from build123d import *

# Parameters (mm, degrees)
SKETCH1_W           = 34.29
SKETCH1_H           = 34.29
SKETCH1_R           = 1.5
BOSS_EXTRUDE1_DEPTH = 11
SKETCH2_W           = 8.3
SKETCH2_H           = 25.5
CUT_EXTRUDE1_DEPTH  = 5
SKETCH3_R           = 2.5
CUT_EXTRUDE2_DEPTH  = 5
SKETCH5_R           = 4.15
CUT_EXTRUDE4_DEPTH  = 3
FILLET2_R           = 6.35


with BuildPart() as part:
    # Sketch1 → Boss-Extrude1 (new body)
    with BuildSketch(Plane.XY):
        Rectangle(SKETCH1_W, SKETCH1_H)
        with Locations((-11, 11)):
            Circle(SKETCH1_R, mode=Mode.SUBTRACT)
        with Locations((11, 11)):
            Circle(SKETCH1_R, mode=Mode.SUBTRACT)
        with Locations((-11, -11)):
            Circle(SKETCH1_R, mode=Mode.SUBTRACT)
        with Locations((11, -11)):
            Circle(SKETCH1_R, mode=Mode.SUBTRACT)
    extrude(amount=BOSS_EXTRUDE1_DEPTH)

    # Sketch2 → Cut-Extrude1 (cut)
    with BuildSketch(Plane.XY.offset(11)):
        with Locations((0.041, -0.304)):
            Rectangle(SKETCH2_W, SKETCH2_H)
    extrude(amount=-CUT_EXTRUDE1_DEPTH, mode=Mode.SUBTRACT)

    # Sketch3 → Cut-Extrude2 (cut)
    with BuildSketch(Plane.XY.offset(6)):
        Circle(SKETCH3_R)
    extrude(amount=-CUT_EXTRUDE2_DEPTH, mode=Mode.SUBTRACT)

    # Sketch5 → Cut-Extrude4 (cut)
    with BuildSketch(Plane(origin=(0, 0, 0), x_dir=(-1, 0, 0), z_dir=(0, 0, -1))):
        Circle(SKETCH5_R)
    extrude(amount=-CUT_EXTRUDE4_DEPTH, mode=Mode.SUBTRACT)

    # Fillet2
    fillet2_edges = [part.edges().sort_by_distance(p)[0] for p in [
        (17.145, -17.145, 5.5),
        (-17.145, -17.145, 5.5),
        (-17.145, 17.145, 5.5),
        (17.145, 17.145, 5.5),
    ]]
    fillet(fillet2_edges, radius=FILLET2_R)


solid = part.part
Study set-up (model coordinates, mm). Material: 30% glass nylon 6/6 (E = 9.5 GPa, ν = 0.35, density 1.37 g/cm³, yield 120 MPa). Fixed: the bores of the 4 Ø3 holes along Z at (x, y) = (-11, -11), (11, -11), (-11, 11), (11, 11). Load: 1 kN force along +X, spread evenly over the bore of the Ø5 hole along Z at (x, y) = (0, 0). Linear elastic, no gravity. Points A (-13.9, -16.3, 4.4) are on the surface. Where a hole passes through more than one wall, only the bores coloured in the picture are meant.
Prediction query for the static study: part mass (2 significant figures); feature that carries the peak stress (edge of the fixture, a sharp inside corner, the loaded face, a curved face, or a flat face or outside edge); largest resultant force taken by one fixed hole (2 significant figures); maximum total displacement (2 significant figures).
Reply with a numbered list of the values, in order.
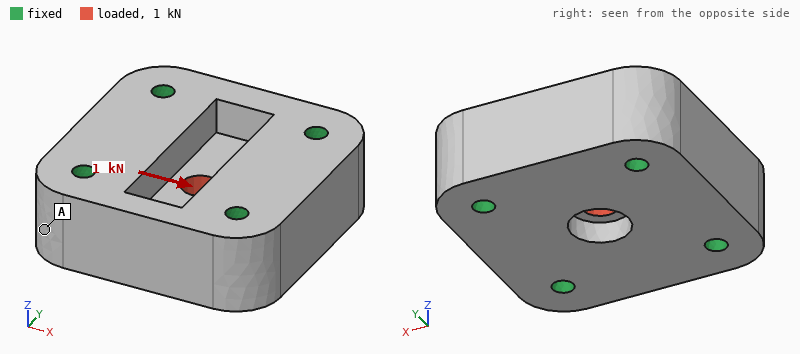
1. 15 g
2. the loaded face
3. 270 N
4. 13 µm
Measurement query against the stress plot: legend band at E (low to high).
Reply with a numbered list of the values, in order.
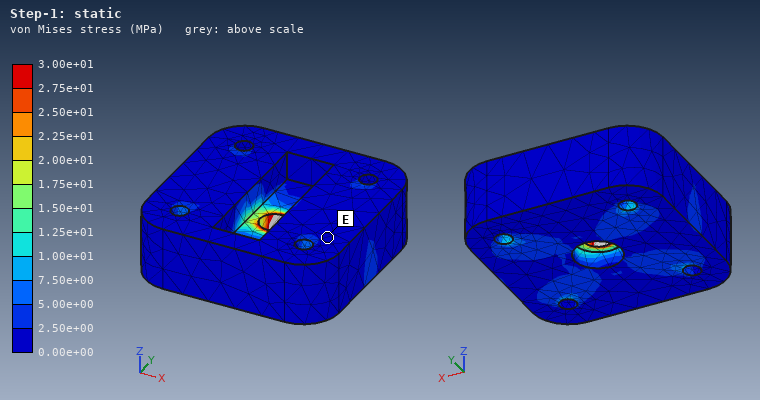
1. 0.00e+00 to 2.50e+00 MPa
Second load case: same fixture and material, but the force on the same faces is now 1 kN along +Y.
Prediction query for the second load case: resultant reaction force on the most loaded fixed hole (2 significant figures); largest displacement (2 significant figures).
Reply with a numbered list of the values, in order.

1. 270 N
2. 15 µm
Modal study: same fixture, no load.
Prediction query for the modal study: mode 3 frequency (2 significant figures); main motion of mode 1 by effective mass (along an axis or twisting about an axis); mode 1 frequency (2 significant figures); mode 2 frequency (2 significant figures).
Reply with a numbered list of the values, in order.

1. 29 kHz
2. along Z
3. 24 kHz
4. 29 kHz
